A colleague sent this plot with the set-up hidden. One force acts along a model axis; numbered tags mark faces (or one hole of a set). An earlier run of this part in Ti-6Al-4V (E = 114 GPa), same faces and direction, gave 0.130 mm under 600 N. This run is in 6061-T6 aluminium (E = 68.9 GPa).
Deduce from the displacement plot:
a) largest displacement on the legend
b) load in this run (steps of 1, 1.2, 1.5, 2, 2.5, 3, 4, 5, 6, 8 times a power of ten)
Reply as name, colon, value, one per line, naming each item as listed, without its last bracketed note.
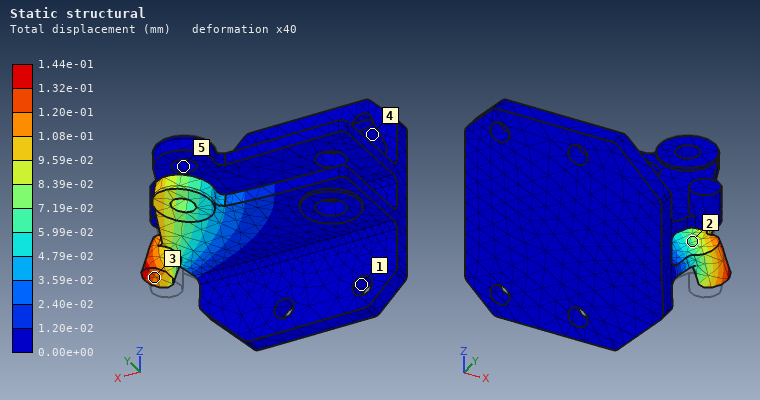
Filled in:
largest displacement on the legend: 1.44e-01 mm
load in this run: 400 N
